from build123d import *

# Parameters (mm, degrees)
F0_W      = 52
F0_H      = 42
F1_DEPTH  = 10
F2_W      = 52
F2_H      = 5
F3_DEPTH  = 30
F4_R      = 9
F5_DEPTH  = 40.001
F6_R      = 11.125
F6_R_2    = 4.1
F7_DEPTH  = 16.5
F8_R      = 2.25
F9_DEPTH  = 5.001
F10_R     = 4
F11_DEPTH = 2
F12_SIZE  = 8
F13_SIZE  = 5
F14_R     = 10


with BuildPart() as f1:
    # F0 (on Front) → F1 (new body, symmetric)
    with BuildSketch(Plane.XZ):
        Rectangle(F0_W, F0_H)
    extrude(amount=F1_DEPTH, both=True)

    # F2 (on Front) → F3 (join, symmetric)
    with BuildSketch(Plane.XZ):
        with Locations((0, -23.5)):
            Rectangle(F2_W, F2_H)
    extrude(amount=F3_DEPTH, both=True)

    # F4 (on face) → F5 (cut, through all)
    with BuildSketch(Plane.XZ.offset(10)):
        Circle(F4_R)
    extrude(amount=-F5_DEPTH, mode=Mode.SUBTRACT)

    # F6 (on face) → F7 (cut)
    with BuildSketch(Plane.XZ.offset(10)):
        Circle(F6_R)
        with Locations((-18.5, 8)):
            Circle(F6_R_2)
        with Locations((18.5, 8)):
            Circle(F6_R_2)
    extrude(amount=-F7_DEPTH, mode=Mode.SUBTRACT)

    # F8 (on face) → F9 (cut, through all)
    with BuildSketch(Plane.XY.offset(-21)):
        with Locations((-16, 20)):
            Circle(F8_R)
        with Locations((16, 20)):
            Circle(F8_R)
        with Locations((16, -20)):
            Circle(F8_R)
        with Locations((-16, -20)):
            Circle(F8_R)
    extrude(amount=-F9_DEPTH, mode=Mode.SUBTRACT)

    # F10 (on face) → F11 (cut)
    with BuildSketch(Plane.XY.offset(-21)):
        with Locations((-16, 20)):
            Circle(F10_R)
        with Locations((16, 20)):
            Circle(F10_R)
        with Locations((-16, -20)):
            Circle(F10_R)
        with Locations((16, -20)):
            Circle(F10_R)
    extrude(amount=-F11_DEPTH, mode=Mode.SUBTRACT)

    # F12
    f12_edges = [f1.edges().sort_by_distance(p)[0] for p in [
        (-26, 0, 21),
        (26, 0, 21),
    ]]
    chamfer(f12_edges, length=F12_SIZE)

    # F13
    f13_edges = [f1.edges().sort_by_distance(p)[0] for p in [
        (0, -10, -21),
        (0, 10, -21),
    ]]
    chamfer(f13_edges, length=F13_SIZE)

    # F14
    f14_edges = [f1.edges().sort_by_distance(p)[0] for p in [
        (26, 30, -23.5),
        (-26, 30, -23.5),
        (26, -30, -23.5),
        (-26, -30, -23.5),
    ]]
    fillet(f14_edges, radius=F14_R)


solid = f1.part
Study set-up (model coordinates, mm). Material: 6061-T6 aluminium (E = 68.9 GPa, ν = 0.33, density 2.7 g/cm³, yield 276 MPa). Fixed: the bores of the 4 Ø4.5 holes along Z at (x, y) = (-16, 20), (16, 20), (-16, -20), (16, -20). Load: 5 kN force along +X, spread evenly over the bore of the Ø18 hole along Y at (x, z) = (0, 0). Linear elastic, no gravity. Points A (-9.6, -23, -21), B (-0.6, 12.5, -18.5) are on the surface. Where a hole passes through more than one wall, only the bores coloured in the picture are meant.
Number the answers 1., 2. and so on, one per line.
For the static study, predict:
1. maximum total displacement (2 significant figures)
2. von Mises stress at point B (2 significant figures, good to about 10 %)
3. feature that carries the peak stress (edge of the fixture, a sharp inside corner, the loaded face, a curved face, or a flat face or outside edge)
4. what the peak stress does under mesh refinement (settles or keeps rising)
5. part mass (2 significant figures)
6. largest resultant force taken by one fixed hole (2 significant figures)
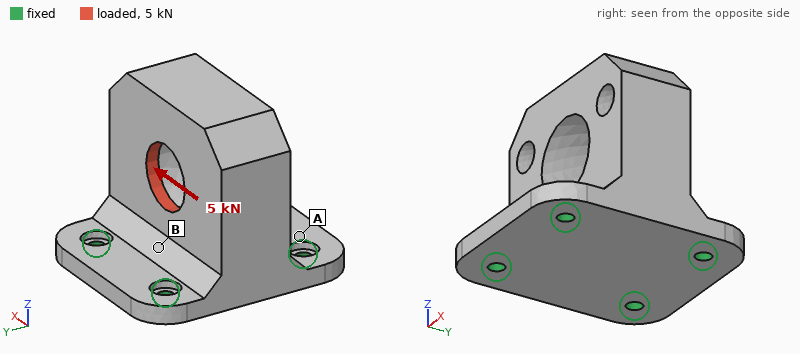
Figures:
1. 86 µm
2. 41 MPa
3. edge of the fixture
4. keeps rising
5. 130 g
6. 2.9 kN
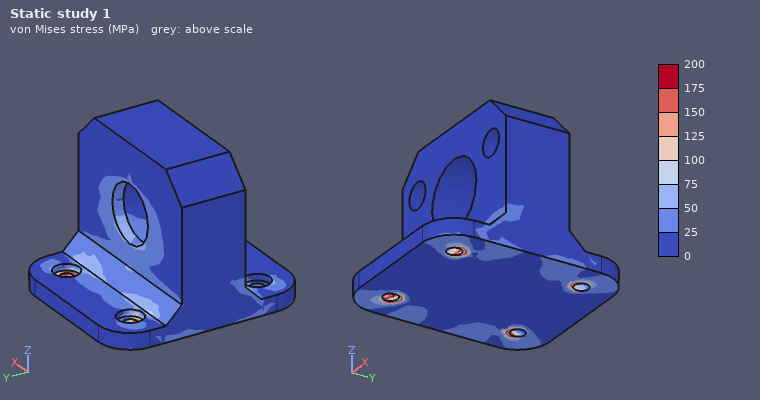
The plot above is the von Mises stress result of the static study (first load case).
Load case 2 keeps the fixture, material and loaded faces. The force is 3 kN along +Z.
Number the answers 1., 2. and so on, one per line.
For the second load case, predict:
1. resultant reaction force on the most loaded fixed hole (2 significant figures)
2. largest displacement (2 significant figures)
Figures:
1. 1.2 kN
2. 25 µm
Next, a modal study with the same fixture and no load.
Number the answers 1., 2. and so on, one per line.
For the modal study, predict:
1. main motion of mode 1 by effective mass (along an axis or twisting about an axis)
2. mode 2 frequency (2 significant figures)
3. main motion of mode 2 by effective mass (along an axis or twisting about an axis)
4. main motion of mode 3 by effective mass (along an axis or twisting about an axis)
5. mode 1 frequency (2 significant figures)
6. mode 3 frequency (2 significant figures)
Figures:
1. along X
2. 5300 Hz
3. along Y
4. along Z
5. 4600 Hz
6. 8600 Hz
